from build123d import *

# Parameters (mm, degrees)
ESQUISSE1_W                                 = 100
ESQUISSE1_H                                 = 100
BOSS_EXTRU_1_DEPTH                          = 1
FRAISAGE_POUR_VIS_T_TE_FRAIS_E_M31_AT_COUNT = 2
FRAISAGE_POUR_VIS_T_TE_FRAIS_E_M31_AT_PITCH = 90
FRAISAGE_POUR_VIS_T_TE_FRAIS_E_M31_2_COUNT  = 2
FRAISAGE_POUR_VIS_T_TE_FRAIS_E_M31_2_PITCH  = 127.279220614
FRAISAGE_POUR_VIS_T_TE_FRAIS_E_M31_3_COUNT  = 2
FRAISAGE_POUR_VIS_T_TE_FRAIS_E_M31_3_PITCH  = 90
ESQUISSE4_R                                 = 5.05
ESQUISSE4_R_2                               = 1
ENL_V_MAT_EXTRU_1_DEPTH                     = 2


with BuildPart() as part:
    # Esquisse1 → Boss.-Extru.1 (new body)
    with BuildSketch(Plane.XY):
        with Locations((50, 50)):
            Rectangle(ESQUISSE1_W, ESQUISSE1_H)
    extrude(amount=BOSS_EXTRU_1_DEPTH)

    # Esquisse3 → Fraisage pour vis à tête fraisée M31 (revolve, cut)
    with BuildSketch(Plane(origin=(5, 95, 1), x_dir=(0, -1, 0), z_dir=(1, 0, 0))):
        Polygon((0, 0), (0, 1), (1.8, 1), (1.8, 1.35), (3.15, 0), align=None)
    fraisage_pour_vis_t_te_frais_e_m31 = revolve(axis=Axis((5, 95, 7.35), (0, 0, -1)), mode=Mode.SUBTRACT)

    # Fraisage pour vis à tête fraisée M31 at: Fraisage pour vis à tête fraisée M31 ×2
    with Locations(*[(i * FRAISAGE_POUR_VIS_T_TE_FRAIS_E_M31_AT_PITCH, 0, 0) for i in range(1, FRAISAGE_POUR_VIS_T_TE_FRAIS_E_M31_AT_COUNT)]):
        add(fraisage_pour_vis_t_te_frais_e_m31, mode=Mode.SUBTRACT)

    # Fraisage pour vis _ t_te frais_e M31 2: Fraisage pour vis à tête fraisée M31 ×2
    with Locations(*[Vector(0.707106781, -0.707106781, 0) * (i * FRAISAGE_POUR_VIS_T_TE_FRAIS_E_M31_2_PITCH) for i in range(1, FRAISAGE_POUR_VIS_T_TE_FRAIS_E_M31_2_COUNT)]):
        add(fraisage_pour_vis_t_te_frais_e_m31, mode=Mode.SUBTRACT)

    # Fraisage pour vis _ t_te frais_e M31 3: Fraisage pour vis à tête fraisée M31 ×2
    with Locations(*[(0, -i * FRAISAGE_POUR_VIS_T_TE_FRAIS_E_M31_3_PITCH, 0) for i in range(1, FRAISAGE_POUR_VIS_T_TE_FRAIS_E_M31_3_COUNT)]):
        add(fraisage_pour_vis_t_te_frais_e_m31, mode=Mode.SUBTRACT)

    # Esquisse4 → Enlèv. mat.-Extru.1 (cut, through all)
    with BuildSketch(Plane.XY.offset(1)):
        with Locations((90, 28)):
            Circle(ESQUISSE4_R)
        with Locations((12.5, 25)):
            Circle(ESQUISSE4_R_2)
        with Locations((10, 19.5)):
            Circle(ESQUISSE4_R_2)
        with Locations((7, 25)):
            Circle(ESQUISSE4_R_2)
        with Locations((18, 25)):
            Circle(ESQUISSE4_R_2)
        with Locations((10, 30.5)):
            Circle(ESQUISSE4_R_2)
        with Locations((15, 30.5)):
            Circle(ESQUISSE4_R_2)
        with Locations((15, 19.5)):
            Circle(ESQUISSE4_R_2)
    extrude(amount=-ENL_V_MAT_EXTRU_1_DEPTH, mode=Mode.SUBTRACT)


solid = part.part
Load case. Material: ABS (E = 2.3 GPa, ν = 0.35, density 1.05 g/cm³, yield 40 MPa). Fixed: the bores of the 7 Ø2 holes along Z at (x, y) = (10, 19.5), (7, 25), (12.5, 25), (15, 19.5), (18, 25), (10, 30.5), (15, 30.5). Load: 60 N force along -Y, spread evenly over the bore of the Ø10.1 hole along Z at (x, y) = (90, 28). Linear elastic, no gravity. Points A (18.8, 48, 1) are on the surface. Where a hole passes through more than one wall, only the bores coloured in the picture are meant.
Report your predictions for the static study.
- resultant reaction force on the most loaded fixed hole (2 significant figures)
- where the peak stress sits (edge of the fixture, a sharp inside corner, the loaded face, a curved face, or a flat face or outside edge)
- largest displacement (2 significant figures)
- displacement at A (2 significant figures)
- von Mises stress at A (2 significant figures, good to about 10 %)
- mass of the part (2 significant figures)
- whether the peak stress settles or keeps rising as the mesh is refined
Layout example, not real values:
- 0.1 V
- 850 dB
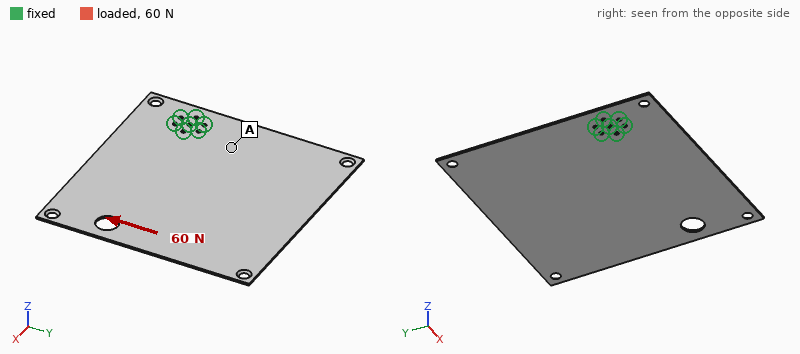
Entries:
- 140 N
- edge of the fixture
- 1.6 mm
- 0.29 mm
- 3.9 MPa
- 10 g
- keeps rising
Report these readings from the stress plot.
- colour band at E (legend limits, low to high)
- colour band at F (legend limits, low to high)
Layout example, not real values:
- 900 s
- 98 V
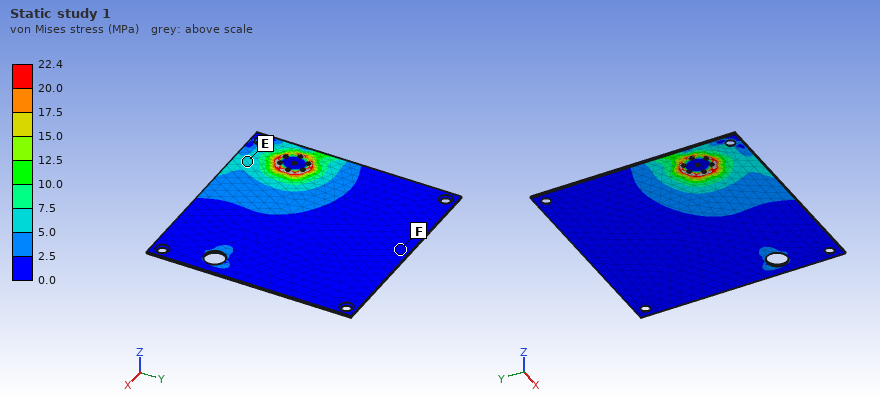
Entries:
- 5.0 to 7.5 MPa
- 0.0 to 2.5 MPa
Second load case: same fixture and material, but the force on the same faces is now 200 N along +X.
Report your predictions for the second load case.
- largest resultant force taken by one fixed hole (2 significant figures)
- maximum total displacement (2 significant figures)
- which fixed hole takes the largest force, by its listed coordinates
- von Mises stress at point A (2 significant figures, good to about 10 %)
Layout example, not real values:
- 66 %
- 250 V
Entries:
- 66 N
- 0.27 mm
- (15, 30.5)
- 2.0 MPa
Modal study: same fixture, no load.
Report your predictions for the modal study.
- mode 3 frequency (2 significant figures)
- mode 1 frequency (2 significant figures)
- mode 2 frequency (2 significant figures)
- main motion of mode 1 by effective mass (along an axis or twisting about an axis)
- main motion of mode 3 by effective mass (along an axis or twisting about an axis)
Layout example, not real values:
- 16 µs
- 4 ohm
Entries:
- 92 Hz
- 25 Hz
- 43 Hz
- along Z
- along Z
